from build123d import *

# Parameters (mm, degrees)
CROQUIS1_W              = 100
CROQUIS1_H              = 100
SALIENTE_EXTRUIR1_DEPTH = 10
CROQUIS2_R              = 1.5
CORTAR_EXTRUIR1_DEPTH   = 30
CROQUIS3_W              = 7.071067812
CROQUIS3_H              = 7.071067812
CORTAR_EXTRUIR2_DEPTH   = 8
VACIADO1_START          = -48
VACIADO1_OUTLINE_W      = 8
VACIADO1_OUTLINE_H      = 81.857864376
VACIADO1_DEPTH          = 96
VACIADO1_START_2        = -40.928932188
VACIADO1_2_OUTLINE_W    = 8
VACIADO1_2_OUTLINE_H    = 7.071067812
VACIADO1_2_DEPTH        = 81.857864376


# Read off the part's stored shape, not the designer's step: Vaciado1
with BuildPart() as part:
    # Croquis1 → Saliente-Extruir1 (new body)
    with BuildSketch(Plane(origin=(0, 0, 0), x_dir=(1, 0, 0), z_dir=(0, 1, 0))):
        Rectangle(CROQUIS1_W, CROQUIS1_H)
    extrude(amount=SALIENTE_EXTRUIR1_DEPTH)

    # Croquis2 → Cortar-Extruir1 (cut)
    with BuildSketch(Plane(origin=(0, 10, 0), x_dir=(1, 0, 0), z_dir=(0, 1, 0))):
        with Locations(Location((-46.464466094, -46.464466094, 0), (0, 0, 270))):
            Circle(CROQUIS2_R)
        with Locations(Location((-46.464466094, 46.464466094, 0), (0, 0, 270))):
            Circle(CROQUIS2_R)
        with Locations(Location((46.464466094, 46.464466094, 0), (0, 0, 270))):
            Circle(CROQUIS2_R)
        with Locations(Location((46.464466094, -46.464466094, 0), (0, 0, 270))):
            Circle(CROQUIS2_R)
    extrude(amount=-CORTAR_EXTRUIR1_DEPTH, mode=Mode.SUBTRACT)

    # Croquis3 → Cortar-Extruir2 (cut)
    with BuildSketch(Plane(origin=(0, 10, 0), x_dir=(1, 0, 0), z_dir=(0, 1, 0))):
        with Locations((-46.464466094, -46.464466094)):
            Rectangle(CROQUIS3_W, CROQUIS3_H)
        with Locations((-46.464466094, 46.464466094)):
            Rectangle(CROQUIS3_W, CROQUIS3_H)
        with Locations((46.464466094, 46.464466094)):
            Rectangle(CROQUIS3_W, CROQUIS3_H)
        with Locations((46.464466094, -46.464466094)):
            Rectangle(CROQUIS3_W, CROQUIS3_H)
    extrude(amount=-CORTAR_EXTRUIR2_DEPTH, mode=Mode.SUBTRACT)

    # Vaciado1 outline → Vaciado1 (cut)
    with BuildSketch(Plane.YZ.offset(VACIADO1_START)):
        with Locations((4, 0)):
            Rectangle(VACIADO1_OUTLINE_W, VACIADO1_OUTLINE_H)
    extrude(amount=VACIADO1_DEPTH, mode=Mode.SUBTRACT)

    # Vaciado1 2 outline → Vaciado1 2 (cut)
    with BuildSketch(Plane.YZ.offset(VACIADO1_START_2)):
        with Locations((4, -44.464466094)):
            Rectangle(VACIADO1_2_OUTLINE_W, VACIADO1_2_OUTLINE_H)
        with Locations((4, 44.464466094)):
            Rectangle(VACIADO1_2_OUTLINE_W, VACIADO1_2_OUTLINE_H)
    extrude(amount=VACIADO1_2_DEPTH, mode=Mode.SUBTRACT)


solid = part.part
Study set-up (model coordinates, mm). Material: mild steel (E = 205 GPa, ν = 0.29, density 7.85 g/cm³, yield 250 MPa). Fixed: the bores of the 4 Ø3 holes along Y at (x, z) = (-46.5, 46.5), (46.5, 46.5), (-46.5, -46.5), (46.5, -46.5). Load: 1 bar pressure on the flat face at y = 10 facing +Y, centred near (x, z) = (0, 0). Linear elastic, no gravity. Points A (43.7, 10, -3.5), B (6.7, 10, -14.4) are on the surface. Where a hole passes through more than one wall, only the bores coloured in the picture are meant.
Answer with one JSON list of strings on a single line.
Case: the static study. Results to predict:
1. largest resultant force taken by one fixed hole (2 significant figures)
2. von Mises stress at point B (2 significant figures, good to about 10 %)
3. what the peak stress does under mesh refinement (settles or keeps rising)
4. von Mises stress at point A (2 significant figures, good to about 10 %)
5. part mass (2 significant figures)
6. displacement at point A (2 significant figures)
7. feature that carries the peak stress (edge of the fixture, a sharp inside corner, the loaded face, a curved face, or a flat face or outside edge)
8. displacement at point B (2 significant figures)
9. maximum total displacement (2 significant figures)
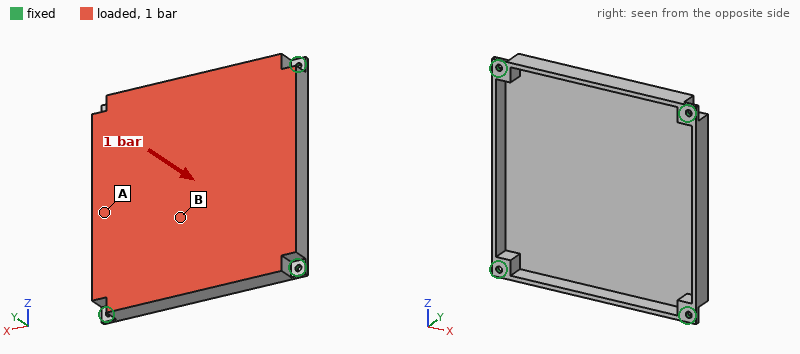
["530 N", "50 MPa", "keeps rising", "20 MPa", "210 g", "0.038 mm", "edge of the fixture", "0.16 mm", "0.18 mm"]
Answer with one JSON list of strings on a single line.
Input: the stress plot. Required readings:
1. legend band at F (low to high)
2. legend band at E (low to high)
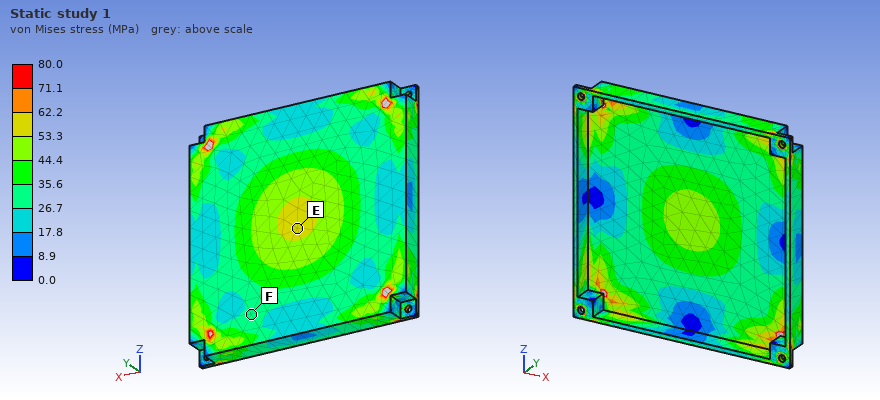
["26.7 to 35.6 MPa", "53.3 to 62.2 MPa"]
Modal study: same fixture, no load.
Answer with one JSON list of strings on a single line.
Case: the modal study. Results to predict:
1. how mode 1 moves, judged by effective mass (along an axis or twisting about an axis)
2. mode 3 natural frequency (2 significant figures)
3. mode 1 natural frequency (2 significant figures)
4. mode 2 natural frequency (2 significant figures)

["along Y", "2600 Hz", "1200 Hz", "2600 Hz"]
